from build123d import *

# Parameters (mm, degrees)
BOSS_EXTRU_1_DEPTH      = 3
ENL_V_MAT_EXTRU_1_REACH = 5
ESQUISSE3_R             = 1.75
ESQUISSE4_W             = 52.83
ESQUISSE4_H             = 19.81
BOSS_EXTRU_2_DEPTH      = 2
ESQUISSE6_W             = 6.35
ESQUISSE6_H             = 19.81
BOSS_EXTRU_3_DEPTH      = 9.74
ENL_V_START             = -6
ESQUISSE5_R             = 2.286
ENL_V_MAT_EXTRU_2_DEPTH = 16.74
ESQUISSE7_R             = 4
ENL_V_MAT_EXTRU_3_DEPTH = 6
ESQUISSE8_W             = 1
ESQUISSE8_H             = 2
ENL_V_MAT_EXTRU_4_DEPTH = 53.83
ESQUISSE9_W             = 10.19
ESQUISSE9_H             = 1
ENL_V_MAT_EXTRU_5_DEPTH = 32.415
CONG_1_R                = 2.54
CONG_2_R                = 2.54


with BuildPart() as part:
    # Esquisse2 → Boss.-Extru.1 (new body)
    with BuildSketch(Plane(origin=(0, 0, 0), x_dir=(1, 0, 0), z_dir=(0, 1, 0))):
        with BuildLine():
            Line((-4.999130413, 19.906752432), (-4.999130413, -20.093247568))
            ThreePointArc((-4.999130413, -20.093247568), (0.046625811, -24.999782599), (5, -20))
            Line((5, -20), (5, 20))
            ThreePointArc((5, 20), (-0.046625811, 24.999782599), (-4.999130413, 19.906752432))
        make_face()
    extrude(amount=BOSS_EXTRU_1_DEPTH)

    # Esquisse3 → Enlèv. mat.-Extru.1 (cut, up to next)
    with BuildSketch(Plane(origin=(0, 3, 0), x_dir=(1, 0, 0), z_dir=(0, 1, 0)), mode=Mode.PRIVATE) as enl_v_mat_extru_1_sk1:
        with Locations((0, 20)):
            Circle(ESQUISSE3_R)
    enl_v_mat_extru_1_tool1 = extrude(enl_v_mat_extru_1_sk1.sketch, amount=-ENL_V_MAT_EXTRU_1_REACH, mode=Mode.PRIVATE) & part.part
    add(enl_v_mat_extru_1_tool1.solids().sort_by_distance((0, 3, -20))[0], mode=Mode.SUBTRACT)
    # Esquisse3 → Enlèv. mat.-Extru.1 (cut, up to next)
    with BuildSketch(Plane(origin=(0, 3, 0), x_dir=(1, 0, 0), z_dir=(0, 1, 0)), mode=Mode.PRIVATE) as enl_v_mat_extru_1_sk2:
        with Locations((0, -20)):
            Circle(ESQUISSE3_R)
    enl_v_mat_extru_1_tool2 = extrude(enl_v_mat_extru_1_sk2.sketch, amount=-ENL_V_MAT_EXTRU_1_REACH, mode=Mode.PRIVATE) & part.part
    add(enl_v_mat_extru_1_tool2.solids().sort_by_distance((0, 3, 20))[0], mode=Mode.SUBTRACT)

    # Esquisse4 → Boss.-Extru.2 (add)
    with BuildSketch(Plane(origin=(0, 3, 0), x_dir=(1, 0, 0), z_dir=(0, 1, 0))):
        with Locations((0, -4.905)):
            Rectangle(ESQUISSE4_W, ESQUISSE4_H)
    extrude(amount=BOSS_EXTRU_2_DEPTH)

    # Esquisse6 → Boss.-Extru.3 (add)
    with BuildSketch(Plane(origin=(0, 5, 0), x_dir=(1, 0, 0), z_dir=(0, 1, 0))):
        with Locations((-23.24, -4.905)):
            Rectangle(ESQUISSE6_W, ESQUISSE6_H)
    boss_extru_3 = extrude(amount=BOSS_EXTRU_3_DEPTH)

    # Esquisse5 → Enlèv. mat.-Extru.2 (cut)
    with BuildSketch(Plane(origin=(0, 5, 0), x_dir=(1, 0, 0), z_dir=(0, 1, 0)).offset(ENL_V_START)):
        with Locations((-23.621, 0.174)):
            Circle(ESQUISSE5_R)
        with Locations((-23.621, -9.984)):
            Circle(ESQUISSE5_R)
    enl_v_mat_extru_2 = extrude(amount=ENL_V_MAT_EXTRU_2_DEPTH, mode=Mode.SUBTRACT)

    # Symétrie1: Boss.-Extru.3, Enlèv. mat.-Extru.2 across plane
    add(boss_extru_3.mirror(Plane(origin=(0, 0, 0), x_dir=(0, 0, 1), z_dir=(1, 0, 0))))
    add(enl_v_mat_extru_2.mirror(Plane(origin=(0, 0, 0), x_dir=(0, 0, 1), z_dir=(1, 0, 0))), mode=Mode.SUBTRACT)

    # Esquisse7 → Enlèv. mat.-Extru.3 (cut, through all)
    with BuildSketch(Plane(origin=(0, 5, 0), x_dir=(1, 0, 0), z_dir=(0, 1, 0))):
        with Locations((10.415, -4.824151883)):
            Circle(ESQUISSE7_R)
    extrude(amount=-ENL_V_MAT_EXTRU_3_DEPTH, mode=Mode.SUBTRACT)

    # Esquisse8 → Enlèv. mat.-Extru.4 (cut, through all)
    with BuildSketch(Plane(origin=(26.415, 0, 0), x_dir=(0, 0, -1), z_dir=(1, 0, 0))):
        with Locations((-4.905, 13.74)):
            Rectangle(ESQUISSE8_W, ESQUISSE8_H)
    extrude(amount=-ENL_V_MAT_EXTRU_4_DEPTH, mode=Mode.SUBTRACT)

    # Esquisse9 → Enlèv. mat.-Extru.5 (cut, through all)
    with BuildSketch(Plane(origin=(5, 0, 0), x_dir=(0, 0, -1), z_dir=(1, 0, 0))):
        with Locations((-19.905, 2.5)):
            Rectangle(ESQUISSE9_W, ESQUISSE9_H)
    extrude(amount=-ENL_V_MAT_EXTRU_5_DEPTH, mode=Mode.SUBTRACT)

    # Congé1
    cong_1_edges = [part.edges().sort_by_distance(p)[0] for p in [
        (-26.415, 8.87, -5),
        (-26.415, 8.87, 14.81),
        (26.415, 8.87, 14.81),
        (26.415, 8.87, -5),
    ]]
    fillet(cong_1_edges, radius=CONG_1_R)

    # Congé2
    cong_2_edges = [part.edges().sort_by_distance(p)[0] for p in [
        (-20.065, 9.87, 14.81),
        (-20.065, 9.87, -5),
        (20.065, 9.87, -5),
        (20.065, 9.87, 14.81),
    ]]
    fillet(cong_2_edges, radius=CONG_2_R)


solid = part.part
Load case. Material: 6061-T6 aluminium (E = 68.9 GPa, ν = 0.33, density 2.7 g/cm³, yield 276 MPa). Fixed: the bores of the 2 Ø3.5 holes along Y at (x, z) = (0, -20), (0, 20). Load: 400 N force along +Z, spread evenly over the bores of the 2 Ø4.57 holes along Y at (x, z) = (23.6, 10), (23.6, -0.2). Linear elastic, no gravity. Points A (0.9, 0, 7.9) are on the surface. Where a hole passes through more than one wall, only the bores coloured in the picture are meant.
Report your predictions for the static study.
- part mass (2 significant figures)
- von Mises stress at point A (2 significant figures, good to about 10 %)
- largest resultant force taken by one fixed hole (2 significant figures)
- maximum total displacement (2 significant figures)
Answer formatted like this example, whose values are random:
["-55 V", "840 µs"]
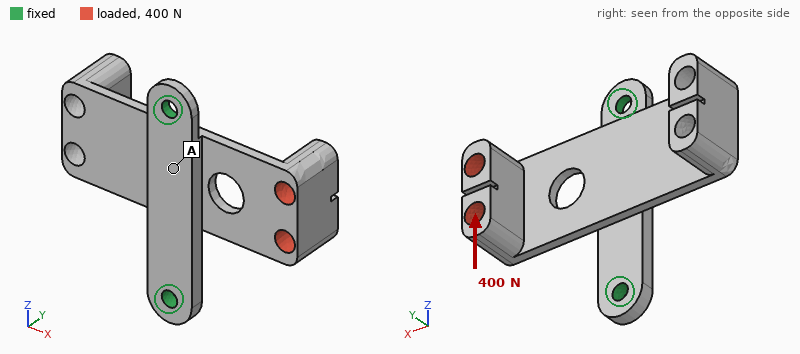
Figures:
["13 g", "16 MPa", "370 N", "0.28 mm"]
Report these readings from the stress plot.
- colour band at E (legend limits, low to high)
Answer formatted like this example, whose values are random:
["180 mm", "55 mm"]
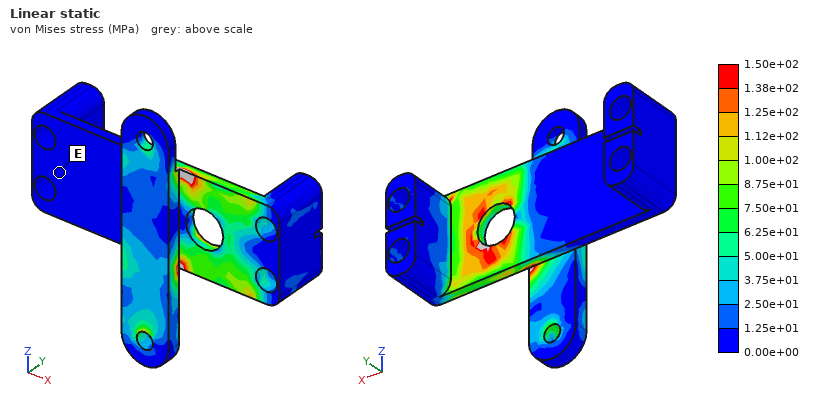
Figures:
["0.00e+00 to 1.25e+01 MPa"]
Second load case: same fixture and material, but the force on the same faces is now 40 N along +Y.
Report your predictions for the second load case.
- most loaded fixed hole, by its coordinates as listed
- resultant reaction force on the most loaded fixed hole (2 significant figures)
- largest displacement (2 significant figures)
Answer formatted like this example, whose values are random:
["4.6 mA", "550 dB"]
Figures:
["(0, 20)", "42 N", "0.31 mm"]
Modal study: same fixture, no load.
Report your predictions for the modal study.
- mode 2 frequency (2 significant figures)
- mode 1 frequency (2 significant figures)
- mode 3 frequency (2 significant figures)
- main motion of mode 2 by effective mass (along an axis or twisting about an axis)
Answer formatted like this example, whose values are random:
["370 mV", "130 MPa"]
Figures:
["1500 Hz", "1100 Hz", "3700 Hz", "along Y"]
